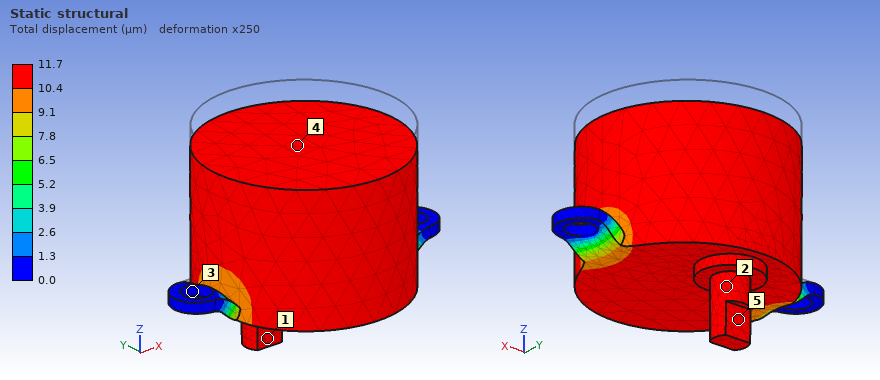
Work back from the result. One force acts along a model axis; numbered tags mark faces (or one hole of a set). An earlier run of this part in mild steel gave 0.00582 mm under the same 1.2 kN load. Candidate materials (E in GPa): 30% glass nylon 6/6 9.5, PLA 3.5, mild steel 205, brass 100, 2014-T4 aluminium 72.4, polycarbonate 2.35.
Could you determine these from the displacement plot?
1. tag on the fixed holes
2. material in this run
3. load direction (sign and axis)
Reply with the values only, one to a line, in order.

3
brass
-Z
